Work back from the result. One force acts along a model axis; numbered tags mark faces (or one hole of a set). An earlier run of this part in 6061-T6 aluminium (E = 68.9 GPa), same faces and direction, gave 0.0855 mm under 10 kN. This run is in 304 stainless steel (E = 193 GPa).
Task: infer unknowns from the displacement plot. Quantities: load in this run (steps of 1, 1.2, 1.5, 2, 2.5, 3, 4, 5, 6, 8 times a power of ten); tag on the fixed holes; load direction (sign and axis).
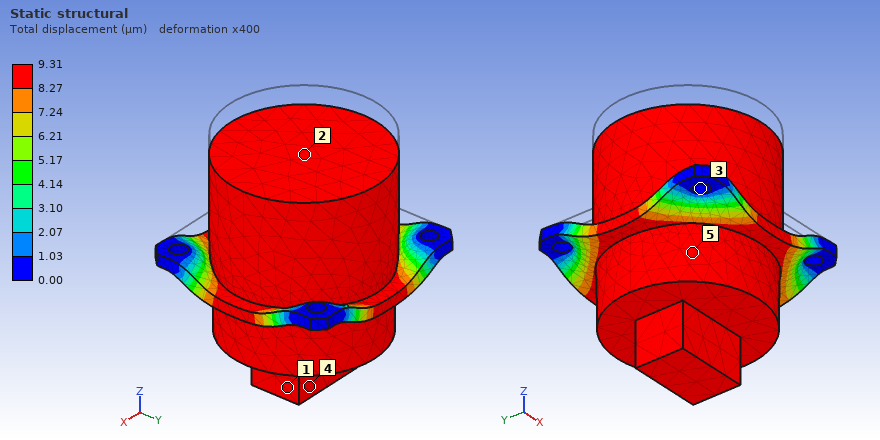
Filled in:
3 kN
3
-Z
